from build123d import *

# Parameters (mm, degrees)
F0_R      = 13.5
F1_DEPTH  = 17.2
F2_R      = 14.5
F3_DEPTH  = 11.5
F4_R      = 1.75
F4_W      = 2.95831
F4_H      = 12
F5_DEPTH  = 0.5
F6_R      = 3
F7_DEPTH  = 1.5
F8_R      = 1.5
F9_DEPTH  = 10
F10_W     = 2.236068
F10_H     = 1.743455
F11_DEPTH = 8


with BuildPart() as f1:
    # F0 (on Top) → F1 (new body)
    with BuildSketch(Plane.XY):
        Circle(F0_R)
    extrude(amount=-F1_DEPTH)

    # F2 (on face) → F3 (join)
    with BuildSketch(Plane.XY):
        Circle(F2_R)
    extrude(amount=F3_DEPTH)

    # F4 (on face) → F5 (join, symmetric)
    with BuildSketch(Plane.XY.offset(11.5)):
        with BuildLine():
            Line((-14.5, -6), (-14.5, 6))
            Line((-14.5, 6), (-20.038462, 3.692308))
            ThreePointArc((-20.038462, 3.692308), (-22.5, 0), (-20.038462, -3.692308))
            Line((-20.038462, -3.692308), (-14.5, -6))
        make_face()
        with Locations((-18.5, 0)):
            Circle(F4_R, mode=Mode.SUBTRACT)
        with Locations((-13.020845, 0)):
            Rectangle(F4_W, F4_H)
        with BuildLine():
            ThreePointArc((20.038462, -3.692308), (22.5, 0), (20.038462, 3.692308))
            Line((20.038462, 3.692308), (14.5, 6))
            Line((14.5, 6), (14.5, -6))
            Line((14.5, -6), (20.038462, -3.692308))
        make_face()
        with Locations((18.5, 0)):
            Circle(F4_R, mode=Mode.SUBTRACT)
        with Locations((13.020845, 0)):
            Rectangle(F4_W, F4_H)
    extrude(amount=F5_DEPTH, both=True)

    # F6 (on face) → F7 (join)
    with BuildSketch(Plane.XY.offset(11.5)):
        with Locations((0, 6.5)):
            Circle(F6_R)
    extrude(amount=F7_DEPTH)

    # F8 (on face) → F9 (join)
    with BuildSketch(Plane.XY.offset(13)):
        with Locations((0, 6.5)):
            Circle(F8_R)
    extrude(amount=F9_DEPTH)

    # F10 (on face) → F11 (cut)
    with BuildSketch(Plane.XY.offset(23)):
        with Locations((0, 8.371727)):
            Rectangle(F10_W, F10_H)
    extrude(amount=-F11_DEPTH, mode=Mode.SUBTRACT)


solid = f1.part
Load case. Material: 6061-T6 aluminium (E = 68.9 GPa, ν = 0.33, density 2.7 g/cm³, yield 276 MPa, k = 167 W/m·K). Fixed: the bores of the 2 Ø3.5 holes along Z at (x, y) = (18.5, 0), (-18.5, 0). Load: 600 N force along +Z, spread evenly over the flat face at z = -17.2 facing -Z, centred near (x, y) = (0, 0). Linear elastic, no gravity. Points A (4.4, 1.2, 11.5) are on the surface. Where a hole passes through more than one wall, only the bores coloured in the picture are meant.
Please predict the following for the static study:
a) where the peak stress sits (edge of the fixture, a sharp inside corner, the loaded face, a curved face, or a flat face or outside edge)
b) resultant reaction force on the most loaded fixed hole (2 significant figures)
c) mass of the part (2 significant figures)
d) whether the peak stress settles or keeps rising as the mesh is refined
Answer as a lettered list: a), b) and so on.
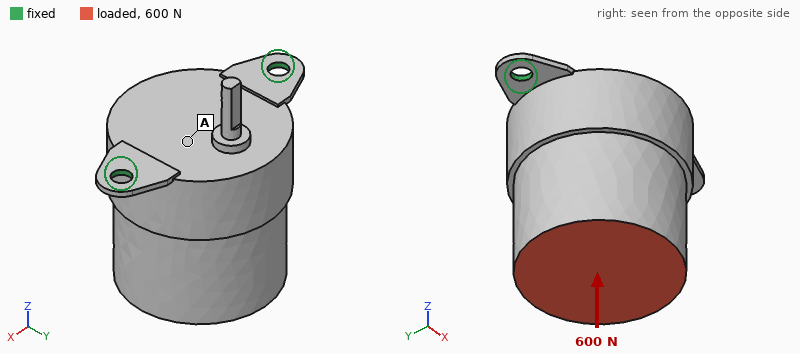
a) edge of the fixture
b) 350 N
c) 48 g
d) keeps rising
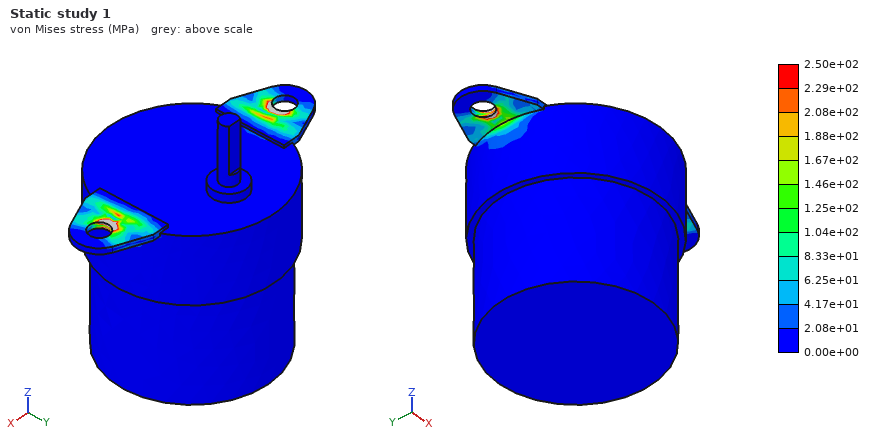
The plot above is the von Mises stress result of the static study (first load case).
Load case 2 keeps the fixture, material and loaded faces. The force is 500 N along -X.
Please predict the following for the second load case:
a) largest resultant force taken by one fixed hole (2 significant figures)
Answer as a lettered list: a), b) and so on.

a) 520 N
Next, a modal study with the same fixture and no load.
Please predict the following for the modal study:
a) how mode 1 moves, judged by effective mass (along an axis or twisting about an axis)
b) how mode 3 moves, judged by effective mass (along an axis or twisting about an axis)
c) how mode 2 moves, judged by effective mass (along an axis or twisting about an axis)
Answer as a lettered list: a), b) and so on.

a) along Y
b) along Z
c) along X
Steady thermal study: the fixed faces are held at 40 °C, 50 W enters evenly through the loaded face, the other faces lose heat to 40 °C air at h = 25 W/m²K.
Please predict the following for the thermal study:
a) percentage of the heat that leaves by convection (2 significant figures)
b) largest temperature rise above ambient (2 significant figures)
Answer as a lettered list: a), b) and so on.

a) 12 %
b) 79 K
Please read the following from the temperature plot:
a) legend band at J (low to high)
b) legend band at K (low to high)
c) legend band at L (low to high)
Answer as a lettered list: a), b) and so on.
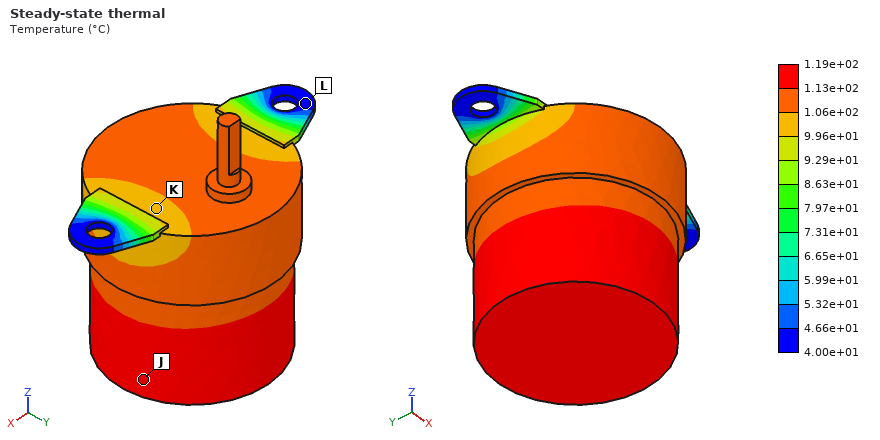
a) 1.13e+02 to 1.19e+02 °C
b) 9.96e+01 to 1.06e+02 °C
c) 4.00e+01 to 4.66e+01 °C
